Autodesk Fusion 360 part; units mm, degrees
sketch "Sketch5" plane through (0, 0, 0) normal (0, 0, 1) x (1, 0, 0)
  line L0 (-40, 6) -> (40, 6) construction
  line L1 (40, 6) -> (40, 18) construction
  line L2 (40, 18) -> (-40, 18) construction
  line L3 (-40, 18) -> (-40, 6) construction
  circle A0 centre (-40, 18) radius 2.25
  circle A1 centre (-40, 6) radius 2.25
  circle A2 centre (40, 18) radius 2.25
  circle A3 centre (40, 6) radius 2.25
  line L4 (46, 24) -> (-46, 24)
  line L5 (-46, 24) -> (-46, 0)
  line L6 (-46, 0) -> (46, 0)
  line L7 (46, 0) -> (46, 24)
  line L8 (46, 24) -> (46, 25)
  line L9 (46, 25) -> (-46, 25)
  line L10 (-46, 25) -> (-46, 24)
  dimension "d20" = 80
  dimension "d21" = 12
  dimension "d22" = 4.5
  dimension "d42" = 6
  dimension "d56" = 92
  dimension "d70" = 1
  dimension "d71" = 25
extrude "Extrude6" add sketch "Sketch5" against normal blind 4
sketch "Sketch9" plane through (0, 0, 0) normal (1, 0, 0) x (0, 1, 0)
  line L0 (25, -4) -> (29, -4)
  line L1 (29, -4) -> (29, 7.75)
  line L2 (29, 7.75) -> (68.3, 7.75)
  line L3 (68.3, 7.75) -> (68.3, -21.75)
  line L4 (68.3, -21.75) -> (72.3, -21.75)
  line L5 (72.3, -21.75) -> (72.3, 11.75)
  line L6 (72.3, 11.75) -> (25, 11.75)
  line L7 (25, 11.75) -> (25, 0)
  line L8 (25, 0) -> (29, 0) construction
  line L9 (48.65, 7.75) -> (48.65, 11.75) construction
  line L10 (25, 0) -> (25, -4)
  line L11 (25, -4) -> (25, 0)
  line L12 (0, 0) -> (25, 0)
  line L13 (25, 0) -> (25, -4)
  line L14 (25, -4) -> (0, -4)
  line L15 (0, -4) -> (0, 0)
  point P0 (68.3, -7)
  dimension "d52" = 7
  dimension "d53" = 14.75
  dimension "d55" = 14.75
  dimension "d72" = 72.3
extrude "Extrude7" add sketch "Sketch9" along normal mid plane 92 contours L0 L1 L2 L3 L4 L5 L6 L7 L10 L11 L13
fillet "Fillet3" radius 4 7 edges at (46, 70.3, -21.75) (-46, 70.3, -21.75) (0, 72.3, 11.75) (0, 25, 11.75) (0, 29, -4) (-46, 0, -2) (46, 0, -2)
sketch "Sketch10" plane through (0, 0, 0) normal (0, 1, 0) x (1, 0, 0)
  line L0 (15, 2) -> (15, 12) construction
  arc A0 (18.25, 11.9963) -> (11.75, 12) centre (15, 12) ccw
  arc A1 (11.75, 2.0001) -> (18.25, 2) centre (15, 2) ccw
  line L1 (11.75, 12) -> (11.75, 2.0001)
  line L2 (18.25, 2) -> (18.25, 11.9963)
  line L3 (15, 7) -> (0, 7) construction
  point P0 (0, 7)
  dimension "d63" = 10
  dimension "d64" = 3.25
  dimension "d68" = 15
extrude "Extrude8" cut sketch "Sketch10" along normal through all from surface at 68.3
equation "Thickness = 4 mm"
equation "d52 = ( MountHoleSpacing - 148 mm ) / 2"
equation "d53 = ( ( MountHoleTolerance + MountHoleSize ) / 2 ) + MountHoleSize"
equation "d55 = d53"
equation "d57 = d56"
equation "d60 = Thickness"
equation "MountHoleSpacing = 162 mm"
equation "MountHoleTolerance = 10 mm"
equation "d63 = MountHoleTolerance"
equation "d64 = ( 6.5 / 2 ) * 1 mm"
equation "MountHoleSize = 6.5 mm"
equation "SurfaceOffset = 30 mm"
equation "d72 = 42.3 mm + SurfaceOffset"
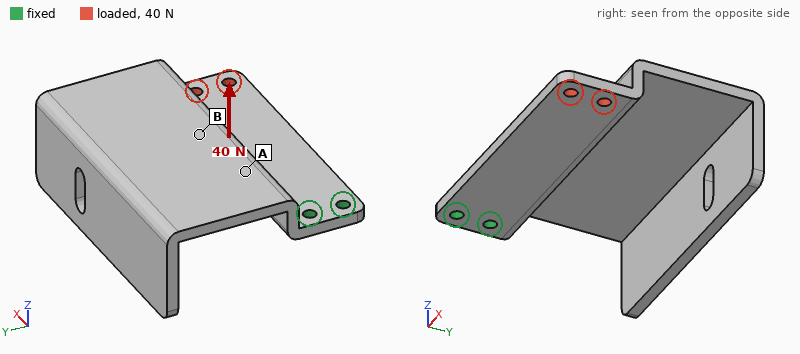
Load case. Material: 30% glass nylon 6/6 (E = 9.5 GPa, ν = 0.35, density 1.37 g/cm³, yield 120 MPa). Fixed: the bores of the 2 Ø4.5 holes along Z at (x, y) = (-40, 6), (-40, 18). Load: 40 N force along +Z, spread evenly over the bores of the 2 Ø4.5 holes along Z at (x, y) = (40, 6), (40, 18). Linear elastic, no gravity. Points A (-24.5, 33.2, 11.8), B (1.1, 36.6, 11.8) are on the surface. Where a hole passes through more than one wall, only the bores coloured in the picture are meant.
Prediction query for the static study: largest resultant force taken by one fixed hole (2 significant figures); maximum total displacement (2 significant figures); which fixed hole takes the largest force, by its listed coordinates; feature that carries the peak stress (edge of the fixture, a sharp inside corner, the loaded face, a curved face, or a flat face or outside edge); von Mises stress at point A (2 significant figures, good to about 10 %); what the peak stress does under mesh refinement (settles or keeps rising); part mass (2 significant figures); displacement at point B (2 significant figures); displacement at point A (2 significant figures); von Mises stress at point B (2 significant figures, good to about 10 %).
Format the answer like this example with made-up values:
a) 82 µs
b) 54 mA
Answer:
a) 43 N
b) 1.3 mm
c) (-40, 18)
d) edge of the fixture
e) 4.6 MPa
f) keeps rising
g) 55 g
h) 0.55 mm
i) 0.24 mm
j) 2.5 MPa
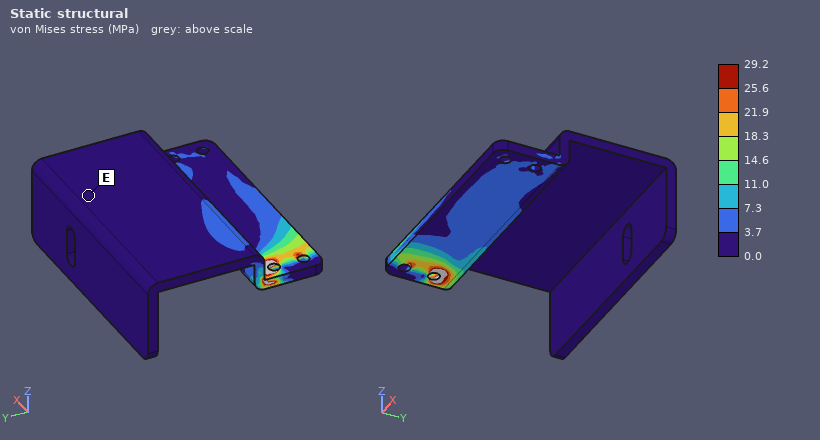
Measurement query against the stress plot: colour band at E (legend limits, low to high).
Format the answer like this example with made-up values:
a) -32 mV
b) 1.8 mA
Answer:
a) 0.0 to 3.7 MPa
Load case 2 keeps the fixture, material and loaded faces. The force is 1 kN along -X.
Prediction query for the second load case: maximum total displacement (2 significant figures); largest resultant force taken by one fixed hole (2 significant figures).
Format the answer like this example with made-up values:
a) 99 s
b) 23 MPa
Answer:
a) 0.15 mm
b) 510 N
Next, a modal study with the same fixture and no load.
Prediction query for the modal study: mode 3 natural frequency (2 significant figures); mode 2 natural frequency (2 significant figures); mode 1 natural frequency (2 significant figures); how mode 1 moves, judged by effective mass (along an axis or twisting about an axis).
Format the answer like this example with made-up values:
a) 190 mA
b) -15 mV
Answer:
a) 450 Hz
b) 330 Hz
c) 150 Hz
d) along Z
